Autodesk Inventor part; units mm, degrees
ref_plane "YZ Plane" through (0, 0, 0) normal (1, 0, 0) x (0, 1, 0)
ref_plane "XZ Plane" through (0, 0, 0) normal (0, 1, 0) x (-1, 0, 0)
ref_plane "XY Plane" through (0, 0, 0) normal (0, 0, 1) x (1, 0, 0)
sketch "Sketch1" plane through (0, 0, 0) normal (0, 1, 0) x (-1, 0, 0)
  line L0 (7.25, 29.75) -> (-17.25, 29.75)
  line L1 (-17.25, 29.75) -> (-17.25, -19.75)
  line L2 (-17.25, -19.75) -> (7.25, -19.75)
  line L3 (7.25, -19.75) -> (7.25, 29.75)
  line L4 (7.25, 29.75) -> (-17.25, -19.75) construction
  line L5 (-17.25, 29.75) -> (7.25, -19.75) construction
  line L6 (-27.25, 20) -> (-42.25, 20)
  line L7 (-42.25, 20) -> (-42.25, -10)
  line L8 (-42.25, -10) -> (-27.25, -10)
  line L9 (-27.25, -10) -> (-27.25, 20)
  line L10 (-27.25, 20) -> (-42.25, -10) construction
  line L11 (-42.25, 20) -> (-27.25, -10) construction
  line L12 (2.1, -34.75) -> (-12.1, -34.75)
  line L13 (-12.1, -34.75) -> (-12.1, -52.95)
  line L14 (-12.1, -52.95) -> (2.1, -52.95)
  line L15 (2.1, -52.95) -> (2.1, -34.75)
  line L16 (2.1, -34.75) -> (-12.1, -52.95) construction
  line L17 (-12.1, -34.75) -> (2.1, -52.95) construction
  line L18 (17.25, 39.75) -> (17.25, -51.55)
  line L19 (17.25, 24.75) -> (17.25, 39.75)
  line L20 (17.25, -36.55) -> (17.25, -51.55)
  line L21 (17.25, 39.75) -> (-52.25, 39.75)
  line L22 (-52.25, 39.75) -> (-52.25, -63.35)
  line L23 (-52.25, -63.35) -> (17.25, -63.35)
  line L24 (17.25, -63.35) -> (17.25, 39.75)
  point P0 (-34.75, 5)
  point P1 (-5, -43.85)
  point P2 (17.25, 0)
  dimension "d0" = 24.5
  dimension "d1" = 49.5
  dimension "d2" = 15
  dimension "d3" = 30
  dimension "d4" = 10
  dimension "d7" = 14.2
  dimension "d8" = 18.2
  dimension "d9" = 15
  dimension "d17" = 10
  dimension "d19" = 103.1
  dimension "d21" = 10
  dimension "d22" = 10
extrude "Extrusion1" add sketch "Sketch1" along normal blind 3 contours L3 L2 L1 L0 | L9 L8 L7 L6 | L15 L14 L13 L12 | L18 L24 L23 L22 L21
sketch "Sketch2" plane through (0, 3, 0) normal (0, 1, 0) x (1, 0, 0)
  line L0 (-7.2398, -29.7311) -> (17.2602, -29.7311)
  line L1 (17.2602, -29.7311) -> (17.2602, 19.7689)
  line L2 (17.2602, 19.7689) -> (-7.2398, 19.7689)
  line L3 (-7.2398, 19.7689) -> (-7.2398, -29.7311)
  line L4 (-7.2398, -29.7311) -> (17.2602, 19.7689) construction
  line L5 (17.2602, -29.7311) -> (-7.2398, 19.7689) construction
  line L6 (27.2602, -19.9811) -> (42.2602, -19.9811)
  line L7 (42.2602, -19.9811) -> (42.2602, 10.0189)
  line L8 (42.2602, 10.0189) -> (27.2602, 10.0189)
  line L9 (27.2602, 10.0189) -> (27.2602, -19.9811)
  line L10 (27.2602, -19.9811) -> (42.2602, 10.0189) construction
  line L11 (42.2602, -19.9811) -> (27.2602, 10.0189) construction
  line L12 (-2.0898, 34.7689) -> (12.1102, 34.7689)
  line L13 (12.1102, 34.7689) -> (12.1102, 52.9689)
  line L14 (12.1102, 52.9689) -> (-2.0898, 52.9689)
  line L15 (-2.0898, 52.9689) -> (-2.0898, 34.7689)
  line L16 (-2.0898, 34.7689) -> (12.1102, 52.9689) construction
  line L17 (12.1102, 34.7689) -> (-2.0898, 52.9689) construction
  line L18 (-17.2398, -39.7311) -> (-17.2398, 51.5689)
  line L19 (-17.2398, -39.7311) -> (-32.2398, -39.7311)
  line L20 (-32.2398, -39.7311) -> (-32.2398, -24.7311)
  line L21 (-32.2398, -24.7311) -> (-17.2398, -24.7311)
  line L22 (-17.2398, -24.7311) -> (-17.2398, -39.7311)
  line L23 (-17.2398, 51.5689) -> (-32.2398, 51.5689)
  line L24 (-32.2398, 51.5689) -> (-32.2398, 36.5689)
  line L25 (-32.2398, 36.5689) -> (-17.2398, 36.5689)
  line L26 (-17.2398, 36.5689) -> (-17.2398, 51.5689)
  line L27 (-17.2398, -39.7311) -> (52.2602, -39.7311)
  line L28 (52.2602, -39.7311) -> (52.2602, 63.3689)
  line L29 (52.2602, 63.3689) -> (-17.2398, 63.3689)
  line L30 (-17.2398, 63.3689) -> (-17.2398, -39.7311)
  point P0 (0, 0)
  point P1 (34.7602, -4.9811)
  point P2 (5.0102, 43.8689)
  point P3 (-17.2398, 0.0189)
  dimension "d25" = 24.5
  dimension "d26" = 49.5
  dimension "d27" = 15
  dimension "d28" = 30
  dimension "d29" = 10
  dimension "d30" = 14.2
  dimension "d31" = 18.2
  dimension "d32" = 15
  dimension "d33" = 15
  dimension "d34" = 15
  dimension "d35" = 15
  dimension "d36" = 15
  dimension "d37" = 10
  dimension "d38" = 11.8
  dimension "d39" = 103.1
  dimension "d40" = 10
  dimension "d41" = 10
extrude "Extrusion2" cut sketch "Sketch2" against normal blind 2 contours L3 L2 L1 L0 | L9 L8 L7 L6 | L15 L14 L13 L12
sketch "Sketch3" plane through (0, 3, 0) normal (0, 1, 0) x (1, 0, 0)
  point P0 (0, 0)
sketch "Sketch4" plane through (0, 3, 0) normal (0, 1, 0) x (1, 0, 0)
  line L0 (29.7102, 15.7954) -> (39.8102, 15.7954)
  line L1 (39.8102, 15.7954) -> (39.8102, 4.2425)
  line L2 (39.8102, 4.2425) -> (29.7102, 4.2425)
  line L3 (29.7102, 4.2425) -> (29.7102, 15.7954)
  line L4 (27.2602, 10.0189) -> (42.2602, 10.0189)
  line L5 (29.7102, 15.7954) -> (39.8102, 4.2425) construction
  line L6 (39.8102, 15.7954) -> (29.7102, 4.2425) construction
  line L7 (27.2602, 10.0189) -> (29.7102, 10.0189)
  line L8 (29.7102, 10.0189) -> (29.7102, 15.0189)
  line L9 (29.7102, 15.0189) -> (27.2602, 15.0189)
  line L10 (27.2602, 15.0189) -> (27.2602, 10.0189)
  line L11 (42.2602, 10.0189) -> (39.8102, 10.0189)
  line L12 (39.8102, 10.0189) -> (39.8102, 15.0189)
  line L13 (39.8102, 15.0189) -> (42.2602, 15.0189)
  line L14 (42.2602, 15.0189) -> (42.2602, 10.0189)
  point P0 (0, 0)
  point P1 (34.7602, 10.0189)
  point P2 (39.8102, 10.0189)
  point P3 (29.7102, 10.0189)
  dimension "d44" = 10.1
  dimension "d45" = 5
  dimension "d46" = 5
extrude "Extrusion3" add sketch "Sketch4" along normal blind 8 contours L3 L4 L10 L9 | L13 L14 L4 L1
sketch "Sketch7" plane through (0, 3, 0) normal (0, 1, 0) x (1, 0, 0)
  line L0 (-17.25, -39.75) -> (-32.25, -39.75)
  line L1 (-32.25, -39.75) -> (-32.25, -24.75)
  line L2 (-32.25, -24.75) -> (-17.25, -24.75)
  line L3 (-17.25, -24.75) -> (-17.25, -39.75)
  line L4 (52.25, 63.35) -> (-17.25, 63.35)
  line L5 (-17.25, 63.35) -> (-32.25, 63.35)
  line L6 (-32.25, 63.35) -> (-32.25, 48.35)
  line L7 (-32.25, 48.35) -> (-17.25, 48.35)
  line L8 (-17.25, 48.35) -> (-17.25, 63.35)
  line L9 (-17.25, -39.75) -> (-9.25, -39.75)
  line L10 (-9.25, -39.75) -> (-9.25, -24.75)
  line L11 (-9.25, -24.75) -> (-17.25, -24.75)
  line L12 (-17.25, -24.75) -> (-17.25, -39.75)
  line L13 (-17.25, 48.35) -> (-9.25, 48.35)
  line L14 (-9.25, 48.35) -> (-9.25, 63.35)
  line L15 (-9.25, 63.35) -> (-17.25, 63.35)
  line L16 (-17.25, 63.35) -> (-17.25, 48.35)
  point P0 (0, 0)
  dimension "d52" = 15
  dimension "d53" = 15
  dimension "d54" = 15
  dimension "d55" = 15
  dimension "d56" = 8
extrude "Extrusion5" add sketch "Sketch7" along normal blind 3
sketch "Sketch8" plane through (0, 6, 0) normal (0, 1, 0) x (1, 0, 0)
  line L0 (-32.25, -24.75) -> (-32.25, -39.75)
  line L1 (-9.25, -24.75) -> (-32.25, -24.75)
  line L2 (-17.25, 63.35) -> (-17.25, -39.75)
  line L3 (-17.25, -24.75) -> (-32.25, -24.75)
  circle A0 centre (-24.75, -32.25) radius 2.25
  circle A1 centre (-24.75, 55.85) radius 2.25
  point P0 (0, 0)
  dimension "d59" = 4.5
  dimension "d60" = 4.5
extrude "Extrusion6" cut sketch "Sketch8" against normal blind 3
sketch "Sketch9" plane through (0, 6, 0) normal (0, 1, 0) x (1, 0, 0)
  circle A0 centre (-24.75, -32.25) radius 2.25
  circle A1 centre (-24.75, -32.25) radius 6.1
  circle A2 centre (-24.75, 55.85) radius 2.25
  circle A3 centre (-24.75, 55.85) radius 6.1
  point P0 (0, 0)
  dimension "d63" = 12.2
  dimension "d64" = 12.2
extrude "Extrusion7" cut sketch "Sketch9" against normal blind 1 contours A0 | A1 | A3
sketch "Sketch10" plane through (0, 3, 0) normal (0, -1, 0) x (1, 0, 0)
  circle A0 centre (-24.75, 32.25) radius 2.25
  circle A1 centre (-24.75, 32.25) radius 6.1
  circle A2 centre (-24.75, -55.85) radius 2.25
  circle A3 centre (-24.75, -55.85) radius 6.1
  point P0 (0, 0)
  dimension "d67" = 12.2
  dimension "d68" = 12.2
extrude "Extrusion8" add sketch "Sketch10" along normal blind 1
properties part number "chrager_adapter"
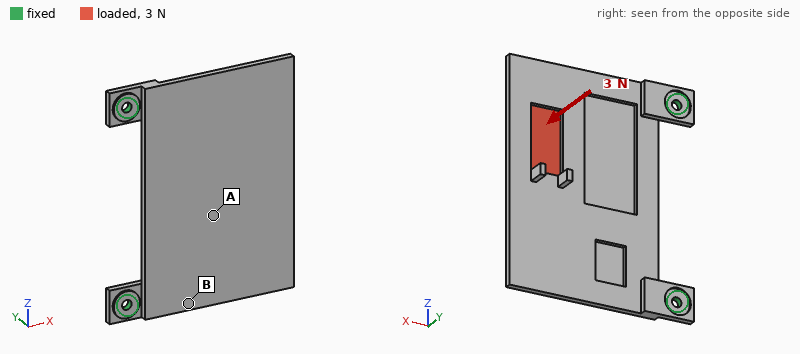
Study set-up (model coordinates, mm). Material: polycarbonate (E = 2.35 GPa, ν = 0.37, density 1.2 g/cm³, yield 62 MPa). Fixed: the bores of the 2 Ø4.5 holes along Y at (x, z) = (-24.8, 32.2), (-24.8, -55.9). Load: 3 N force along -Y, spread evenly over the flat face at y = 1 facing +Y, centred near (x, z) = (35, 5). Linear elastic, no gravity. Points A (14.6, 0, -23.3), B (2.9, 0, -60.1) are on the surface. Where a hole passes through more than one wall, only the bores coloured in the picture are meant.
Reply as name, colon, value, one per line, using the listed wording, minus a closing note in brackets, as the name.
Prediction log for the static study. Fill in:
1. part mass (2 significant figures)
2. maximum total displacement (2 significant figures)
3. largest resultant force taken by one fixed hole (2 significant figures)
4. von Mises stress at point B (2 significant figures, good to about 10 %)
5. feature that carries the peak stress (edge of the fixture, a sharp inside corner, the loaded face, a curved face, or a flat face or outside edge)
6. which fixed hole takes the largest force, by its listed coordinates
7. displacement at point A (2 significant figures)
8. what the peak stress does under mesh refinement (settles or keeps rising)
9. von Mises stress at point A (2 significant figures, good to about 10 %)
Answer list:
part mass: 24 g
maximum total displacement: 1.5 mm
largest resultant force taken by one fixed hole: 2.1 N
von Mises stress at point B: 1.4 MPa
feature that carries the peak stress: edge of the fixture
which fixed hole takes the largest force, by its listed coordinates: (-24.8, 32.2)
displacement at point A: 0.55 mm
what the peak stress does under mesh refinement: keeps rising
von Mises stress at point A: 0.63 MPa
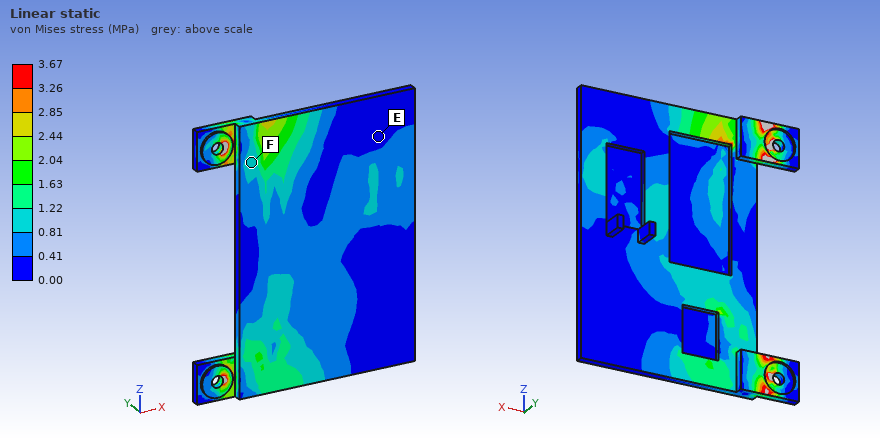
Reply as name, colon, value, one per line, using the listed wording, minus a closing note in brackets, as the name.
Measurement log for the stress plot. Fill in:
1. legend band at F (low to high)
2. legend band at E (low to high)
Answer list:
legend band at F: 0.81 to 1.22 MPa
legend band at E: 0.00 to 0.41 MPa
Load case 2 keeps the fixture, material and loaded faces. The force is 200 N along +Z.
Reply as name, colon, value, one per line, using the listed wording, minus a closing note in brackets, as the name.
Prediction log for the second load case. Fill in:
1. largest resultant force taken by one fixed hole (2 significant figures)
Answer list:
largest resultant force taken by one fixed hole: 160 N
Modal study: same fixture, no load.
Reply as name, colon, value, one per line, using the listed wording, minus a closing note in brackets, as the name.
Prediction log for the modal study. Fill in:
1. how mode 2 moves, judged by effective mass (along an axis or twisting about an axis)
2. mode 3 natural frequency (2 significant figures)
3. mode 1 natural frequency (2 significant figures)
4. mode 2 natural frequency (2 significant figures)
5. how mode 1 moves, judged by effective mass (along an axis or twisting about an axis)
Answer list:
how mode 2 moves, judged by effective mass: twisting about X
mode 3 natural frequency: 460 Hz
mode 1 natural frequency: 77 Hz
mode 2 natural frequency: 200 Hz
how mode 1 moves, judged by effective mass: along Y
